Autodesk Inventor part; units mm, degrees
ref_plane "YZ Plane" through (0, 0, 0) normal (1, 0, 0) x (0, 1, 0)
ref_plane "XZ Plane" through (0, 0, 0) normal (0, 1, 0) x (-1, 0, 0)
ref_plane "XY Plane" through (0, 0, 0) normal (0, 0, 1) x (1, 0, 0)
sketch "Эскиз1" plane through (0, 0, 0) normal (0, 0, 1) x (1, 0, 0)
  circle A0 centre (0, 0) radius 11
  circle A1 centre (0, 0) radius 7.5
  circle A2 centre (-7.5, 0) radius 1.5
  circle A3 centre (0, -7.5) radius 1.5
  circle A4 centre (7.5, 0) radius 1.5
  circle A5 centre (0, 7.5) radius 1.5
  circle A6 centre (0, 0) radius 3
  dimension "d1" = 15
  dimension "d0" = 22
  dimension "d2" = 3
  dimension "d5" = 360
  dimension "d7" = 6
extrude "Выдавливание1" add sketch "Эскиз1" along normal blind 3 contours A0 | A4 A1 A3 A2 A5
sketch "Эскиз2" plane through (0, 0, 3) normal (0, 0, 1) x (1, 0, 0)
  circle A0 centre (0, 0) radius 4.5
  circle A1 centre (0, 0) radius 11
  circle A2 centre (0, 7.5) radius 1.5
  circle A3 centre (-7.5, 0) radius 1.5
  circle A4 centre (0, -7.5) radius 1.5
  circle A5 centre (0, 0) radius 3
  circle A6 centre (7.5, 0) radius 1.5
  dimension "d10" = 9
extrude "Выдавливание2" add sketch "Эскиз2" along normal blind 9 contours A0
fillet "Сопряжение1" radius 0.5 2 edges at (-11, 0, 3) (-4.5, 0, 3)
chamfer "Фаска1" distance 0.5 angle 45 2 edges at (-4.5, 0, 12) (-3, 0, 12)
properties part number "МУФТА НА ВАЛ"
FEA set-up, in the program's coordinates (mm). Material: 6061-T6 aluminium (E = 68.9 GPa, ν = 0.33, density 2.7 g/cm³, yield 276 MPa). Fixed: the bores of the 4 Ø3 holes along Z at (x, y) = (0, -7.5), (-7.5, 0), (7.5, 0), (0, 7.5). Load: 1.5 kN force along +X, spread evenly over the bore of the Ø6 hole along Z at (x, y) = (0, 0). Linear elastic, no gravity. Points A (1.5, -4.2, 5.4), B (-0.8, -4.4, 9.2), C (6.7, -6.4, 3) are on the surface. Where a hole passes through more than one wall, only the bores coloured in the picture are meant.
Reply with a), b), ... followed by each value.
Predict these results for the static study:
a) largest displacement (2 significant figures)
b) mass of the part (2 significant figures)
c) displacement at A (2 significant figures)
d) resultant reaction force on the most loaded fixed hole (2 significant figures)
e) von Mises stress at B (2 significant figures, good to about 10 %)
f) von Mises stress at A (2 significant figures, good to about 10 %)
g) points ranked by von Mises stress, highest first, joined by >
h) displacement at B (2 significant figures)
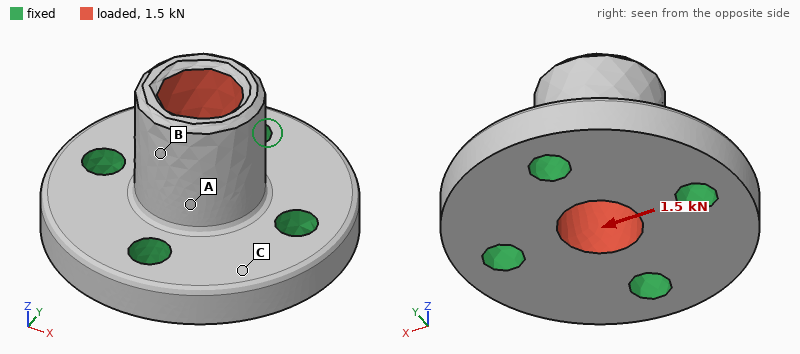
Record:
a) 24 µm
b) 3.5 g
c) 8.1 µm
d) 690 N
e) 27 MPa
f) 49 MPa
g) A > B > C
h) 17 µm
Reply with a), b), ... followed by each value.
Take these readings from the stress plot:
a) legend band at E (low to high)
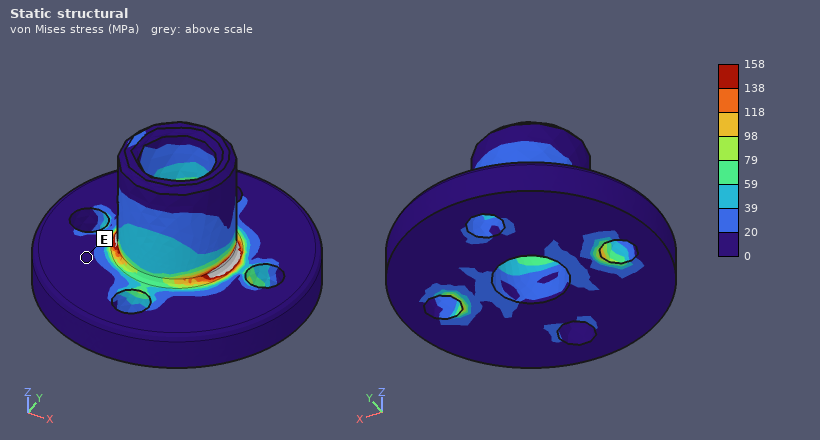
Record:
a) 0 to 20 MPa
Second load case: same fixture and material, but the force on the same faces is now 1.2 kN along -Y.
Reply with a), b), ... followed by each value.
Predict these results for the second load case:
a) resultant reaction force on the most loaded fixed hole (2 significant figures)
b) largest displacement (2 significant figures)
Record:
a) 550 N
b) 19 µm
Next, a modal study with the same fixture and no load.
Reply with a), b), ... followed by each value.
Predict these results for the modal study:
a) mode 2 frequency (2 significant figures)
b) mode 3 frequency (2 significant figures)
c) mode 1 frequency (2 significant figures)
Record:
a) 42 kHz
b) 72 kHz
c) 42 kHz
